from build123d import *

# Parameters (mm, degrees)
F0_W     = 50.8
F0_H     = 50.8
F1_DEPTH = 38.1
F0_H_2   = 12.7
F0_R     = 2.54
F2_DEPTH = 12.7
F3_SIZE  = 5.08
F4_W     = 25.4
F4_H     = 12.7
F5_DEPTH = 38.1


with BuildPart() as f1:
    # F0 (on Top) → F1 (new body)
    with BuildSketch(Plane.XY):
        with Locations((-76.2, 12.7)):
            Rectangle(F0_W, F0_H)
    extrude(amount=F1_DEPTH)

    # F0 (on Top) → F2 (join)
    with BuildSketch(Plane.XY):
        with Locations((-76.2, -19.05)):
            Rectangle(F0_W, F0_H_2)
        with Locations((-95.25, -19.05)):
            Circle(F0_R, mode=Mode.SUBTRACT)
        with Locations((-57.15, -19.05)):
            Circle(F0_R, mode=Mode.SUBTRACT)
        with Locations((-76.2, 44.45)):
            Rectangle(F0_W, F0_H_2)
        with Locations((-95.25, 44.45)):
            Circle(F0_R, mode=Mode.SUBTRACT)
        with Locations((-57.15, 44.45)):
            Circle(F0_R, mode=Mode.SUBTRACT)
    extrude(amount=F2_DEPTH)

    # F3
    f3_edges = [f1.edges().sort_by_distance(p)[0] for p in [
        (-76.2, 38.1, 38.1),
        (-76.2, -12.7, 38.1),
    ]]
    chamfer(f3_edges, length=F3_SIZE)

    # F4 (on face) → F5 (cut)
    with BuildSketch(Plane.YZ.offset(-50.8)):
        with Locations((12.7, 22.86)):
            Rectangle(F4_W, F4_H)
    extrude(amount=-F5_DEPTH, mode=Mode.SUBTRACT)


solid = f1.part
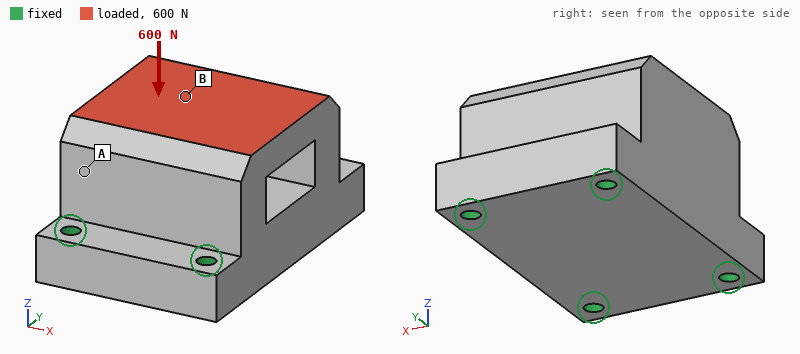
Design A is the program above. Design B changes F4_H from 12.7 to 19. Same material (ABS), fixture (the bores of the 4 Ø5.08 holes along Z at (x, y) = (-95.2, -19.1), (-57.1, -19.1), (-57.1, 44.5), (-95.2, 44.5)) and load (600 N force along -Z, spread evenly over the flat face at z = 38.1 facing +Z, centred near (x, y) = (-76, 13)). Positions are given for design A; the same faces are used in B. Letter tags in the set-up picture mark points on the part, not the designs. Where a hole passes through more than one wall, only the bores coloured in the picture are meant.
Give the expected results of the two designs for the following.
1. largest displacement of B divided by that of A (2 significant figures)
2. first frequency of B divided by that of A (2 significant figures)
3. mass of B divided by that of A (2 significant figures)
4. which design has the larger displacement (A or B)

1.5
1.0
0.94
B
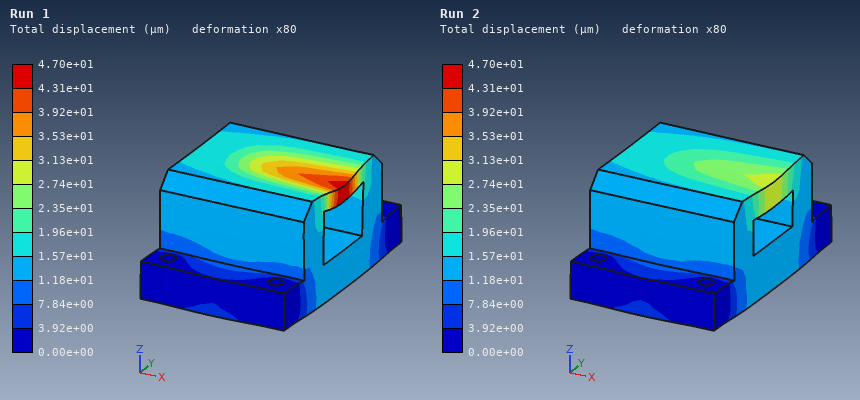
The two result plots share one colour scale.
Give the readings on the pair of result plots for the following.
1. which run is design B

Run 1
